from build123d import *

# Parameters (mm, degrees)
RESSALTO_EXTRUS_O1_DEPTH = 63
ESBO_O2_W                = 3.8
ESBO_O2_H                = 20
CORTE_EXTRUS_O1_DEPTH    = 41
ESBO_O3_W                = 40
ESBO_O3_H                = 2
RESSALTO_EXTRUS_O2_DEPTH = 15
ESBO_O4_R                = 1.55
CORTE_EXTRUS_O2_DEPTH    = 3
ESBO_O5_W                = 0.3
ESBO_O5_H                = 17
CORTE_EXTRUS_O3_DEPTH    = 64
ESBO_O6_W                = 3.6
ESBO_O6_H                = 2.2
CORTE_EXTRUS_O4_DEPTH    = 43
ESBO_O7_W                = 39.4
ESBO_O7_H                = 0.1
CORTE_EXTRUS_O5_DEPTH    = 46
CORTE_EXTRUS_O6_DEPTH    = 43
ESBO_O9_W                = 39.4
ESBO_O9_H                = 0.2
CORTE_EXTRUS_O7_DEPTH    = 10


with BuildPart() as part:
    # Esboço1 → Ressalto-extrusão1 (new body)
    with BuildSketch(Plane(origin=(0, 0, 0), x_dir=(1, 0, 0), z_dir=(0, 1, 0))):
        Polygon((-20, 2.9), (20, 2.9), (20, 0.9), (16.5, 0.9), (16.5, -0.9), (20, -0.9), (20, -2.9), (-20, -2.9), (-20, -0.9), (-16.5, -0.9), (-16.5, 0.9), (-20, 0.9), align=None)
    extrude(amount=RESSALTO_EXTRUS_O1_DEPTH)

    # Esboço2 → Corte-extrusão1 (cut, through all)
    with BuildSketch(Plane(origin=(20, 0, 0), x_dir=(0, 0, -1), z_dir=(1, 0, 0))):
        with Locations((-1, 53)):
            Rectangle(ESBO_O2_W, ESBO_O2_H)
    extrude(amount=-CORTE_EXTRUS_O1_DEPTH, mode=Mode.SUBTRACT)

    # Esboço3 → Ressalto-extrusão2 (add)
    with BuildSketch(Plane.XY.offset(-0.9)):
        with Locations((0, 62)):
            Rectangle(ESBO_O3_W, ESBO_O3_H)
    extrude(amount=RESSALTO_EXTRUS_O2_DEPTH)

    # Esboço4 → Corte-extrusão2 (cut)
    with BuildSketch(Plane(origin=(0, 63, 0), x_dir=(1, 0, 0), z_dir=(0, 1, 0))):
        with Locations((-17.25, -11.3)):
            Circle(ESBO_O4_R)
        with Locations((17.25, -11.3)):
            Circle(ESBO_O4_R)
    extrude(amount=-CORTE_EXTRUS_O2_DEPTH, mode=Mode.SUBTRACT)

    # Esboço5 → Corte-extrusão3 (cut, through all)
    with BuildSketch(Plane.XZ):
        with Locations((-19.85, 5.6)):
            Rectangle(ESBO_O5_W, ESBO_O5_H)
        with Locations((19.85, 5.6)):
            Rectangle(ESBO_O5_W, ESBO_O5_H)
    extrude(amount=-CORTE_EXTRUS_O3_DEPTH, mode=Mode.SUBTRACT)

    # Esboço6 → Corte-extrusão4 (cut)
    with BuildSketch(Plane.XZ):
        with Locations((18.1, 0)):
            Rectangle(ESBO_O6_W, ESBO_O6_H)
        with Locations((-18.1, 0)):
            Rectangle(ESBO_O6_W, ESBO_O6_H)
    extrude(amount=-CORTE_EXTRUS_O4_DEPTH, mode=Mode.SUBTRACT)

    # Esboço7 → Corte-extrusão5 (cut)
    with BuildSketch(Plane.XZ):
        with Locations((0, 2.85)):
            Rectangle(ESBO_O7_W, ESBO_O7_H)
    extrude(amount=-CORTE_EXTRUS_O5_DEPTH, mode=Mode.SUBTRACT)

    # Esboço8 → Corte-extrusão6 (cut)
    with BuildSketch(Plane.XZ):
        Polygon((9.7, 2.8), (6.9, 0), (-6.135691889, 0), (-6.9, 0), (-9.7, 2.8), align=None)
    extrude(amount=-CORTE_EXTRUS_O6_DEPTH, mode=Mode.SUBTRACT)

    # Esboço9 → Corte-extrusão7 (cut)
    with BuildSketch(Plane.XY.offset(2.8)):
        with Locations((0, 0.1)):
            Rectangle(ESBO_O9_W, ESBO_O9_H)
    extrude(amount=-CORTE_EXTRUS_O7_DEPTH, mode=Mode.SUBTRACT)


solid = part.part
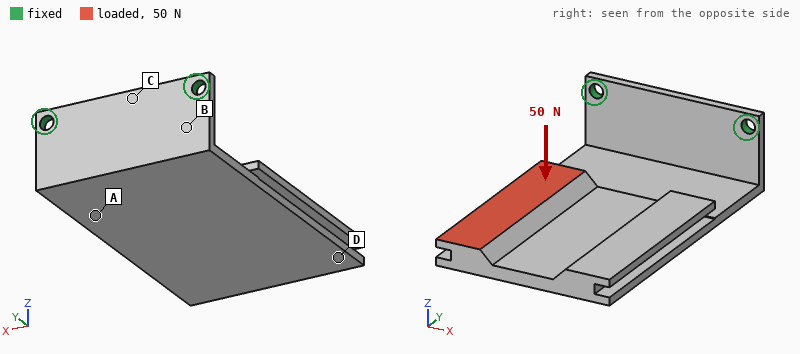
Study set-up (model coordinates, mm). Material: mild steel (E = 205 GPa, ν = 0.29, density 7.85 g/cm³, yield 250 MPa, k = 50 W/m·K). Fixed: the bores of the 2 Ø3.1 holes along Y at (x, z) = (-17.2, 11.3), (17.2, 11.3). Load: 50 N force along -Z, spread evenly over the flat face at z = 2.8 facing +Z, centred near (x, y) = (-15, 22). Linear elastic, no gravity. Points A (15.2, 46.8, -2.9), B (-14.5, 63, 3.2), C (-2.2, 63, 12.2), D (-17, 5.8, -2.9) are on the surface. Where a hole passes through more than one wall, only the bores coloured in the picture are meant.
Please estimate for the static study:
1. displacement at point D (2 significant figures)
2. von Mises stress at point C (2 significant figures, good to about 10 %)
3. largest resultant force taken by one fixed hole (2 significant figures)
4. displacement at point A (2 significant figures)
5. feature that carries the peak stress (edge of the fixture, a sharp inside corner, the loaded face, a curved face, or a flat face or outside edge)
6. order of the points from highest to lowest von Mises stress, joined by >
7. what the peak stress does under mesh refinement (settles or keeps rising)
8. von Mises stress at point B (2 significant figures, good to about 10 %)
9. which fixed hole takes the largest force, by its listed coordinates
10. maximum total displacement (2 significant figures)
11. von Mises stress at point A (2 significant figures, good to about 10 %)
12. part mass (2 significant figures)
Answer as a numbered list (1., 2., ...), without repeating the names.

1. 0.60 mm
2. 29 MPa
3. 52 N
4. 0.12 mm
5. edge of the fixture
6. B > A > C > D
7. keeps rising
8. 87 MPa
9. (-17.2, 11.3)
10. 0.67 mm
11. 54 MPa
12. 76 g
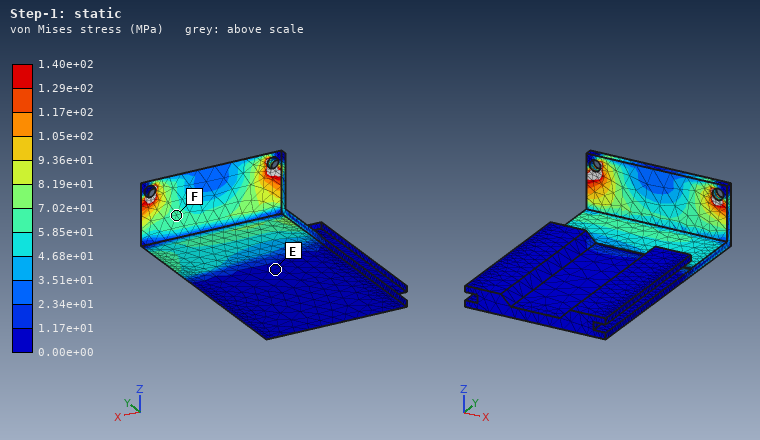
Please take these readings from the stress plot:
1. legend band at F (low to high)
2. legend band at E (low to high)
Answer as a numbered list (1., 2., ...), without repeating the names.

1. 5.85e+01 to 7.02e+01 MPa
2. 0.00e+00 to 1.17e+01 MPa
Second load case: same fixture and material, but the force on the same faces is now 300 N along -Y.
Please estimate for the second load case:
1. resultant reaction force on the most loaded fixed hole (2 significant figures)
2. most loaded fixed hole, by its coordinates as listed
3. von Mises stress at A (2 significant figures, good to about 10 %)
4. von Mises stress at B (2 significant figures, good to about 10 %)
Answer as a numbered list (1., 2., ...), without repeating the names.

1. 280 N
2. (-17.2, 11.3)
3. 39 MPa
4. 83 MPa
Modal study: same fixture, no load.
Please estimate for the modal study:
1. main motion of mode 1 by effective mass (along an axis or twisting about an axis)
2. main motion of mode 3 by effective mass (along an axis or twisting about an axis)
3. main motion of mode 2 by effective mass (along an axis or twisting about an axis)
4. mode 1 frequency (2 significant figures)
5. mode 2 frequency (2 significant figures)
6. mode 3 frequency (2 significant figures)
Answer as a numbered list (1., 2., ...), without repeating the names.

1. along Z
2. along Y
3. along X
4. 230 Hz
5. 730 Hz
6. 1600 Hz
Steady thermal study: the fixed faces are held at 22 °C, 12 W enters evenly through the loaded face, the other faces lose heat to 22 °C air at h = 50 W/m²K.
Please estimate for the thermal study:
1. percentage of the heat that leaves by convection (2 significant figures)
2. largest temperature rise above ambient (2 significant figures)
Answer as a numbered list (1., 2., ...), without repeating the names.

1. 81 %
2. 54 K
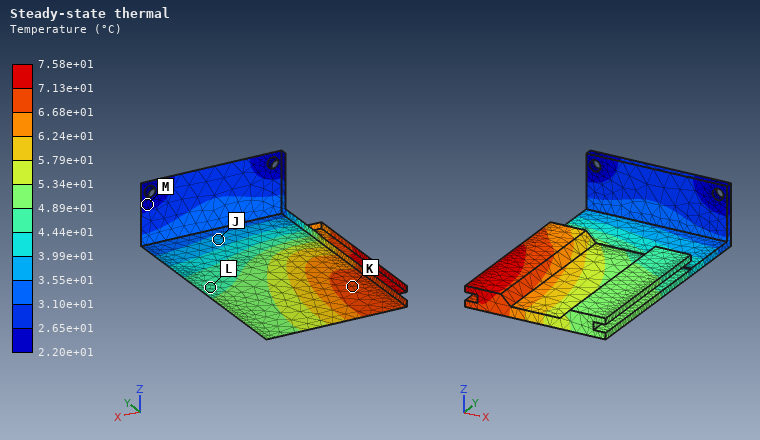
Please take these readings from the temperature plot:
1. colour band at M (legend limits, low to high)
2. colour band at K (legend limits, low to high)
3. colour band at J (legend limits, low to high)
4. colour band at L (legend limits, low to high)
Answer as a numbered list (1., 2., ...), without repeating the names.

1. 2.20e+01 to 2.65e+01 °C
2. 6.68e+01 to 7.13e+01 °C
3. 3.55e+01 to 3.99e+01 °C
4. 4.44e+01 to 4.89e+01 °C
